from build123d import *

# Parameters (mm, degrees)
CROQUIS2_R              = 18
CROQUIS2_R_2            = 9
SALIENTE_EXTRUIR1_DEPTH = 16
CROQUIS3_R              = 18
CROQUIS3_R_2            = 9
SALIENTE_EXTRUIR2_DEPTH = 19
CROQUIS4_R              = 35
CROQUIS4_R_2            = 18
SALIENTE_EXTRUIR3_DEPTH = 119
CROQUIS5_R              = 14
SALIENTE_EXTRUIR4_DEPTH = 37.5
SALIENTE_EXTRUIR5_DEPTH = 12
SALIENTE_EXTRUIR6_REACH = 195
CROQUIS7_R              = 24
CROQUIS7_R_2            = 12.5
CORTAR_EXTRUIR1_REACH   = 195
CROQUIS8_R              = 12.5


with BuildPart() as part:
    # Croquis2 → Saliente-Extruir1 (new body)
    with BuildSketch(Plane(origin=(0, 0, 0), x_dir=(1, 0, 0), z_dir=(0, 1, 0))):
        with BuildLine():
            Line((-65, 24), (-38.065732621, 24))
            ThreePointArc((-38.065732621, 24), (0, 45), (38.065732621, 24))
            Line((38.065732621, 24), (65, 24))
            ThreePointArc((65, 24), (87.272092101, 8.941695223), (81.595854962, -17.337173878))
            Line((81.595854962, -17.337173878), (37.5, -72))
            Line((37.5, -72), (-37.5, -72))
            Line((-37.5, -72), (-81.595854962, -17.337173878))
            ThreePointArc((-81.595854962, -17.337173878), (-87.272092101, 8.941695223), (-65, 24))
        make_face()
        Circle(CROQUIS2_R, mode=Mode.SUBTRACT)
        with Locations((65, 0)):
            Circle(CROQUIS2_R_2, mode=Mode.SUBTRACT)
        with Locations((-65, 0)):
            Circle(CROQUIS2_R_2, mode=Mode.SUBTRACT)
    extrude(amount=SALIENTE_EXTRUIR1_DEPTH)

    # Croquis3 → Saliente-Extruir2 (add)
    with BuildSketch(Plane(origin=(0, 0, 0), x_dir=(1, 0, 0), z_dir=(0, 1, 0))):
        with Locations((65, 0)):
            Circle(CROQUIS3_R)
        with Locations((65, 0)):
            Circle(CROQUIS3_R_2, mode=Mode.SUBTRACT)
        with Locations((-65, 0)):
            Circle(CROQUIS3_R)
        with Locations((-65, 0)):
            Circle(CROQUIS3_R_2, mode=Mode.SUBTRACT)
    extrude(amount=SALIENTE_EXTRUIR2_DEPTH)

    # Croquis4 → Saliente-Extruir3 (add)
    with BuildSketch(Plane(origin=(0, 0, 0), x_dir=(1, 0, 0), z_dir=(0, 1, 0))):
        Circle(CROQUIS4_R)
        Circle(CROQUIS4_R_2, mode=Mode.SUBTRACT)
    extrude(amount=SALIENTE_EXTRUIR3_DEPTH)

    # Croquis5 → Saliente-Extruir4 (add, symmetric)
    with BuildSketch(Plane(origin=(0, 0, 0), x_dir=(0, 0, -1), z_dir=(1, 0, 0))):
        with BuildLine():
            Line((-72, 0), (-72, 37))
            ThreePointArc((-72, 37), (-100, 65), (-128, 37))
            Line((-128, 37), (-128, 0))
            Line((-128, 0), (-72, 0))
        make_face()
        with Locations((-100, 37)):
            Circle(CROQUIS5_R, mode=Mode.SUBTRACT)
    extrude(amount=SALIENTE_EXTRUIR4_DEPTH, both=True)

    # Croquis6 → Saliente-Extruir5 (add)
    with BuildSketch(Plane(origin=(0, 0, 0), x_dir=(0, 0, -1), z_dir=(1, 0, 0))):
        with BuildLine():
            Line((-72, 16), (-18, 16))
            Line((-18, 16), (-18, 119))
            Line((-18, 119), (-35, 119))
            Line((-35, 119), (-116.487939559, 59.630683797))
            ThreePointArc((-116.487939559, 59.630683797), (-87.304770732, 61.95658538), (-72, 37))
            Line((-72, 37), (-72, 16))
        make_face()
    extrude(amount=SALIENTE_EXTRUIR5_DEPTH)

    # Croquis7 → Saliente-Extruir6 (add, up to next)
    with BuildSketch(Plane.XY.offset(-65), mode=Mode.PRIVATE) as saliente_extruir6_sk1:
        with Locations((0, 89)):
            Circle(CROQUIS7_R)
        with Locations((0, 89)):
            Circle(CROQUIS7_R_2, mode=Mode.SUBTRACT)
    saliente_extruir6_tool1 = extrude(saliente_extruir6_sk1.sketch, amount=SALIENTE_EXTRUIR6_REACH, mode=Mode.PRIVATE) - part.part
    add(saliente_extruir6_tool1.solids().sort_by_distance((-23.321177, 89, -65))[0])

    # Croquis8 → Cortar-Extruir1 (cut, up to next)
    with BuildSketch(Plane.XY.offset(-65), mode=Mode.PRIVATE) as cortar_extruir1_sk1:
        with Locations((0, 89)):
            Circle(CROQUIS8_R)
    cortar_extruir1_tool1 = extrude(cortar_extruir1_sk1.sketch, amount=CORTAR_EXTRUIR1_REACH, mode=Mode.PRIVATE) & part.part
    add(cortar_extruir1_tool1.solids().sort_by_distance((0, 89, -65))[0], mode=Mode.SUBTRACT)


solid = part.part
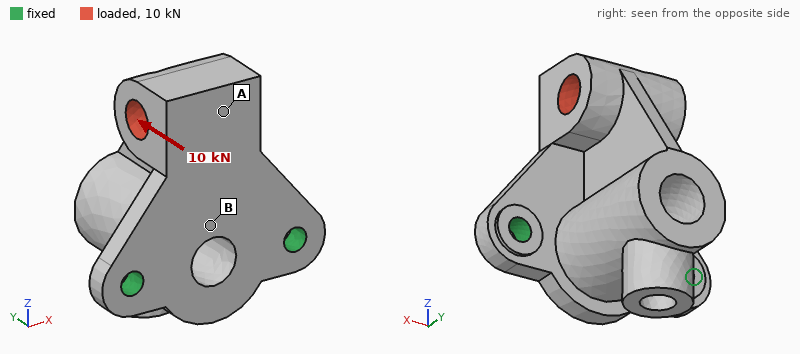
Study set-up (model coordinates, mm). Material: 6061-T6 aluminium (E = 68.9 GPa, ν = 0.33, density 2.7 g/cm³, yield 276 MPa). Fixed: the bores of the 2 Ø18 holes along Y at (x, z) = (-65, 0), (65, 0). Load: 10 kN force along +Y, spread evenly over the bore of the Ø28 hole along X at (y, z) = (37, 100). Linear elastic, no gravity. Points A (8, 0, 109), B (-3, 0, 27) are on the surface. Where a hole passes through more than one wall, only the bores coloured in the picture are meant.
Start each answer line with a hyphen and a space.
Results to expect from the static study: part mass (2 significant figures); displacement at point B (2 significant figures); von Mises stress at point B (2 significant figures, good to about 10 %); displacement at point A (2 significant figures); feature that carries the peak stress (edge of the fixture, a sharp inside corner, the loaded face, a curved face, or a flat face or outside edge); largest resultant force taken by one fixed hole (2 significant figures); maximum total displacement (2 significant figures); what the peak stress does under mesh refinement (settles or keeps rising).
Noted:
- 2.1 kg
- 0.17 mm
- 29 MPa
- 0.65 mm
- edge of the fixture
- 5.1 kN
- 0.79 mm
- keeps rising
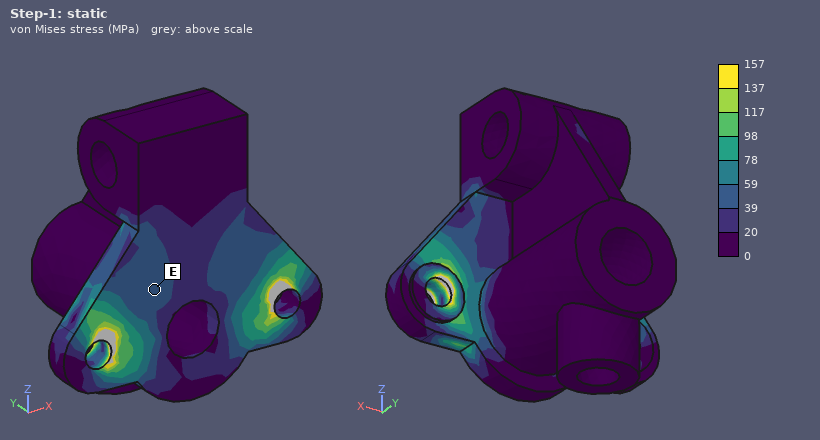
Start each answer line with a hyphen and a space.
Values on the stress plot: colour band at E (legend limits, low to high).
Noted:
- 39 to 59 MPa
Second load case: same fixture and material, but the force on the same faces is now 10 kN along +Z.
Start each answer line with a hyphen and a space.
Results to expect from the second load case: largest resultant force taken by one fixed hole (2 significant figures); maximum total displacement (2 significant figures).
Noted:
- 5.4 kN
- 0.23 mm
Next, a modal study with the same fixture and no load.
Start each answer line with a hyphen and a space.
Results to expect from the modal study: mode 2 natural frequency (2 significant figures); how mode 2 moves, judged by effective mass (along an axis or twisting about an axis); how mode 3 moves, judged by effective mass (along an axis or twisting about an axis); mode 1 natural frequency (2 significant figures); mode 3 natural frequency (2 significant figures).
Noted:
- 1800 Hz
- along X
- along Y
- 600 Hz
- 2400 Hz
